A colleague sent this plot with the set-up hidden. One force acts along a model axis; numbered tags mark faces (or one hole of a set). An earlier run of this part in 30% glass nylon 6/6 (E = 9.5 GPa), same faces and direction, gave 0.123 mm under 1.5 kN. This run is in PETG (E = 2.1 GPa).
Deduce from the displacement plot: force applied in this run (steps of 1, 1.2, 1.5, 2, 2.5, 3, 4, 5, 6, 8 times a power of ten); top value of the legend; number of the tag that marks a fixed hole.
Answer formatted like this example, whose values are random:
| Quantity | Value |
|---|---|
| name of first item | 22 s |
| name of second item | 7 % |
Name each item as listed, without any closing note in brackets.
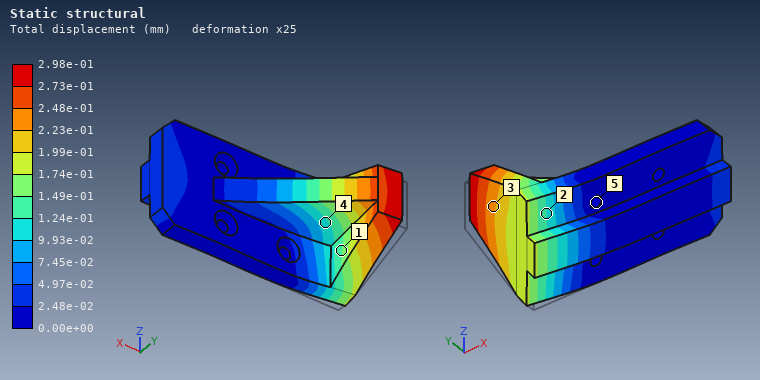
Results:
| Quantity | Value |
|---|---|
| force applied in this run | 800 N |
| top value of the legend | 2.98e-01 mm |
| number of the tag that marks a fixed hole | 5 |
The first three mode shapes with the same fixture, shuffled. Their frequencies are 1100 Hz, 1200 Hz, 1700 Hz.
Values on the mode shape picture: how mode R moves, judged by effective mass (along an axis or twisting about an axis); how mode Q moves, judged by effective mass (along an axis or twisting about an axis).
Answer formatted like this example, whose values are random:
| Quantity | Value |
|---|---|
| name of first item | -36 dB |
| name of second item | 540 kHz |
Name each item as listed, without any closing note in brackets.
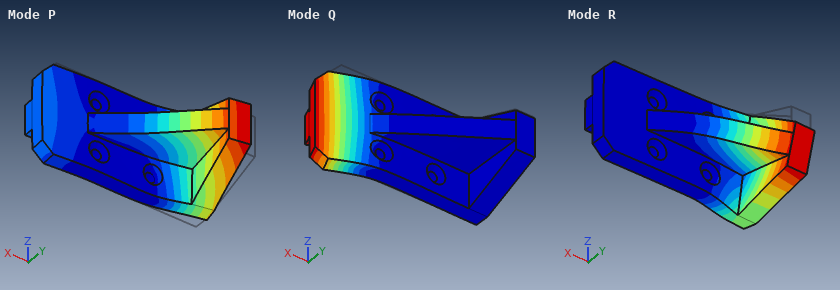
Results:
| Quantity | Value |
|---|---|
| how mode R moves, judged by effective mass | along Z |
| how mode Q moves, judged by effective mass | along Y |
